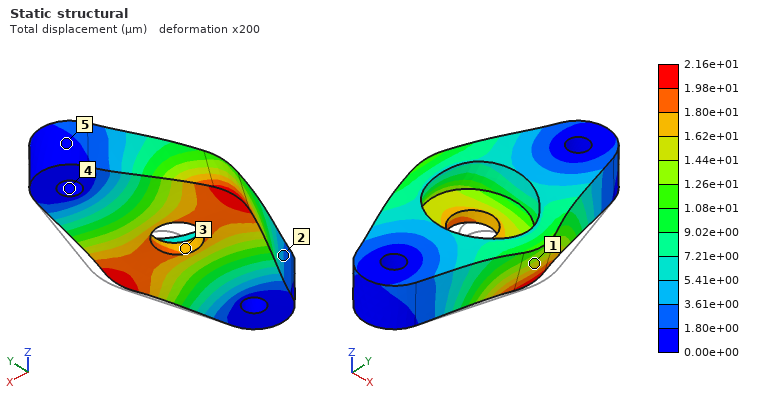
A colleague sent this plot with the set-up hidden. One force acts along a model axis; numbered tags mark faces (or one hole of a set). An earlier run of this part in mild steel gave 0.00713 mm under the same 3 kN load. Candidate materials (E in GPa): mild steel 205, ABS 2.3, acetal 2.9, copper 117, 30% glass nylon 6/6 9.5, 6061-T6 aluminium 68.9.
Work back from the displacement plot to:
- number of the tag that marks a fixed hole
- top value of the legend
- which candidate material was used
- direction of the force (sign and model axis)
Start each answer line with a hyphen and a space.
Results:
- 4
- 2.16e+01 µm
- 6061-T6 aluminium
- -X
